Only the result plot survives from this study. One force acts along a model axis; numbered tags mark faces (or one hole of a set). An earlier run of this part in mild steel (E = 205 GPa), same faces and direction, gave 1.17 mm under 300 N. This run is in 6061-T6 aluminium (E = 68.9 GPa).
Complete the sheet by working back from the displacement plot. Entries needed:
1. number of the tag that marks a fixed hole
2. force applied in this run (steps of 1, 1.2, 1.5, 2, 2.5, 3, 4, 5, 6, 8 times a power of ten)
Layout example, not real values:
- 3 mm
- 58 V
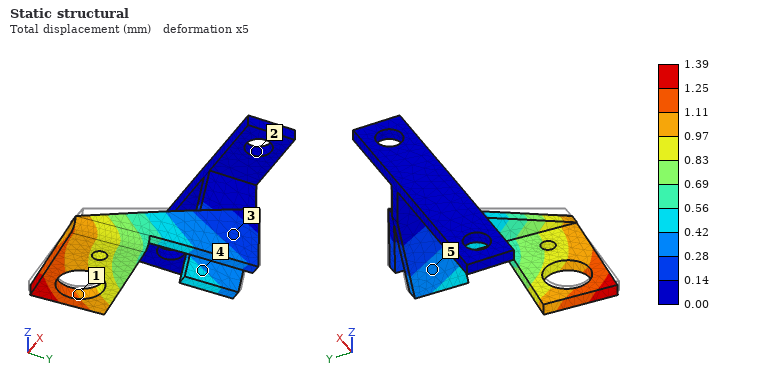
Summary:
- 2
- 120 N
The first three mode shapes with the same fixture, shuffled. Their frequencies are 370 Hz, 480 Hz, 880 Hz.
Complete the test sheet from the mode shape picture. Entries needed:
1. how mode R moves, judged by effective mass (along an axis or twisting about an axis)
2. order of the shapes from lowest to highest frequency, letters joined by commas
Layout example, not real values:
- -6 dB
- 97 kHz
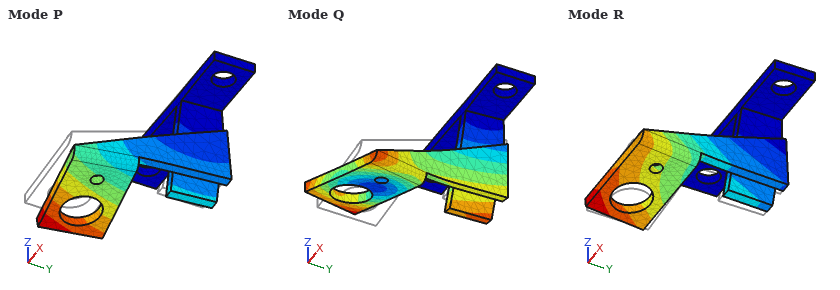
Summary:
- along X
- R, P, Q
